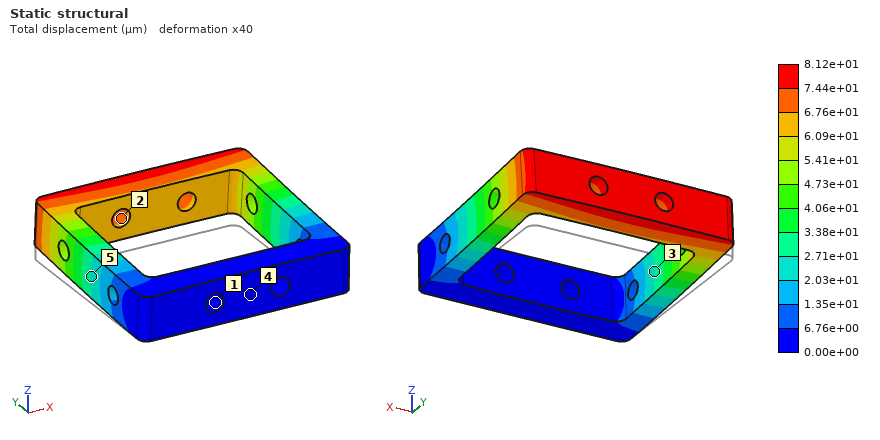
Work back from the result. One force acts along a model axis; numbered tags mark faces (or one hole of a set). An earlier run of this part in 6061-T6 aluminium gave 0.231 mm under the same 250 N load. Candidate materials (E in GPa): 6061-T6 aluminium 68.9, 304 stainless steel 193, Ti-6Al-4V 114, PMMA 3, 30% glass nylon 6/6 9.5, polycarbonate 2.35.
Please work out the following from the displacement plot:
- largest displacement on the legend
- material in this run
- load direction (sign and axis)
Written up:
8.12e+01 µm
304 stainless steel
+Z
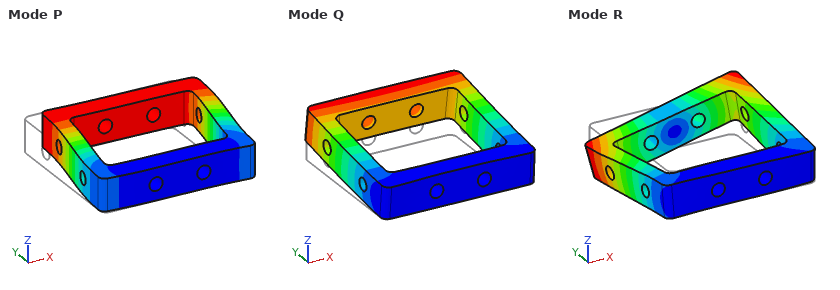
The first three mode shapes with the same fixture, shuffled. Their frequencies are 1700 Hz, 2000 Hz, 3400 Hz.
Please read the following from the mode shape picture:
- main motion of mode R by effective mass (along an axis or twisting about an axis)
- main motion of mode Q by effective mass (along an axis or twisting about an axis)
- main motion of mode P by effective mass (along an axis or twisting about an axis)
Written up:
twisting about Y
along Z
along X
